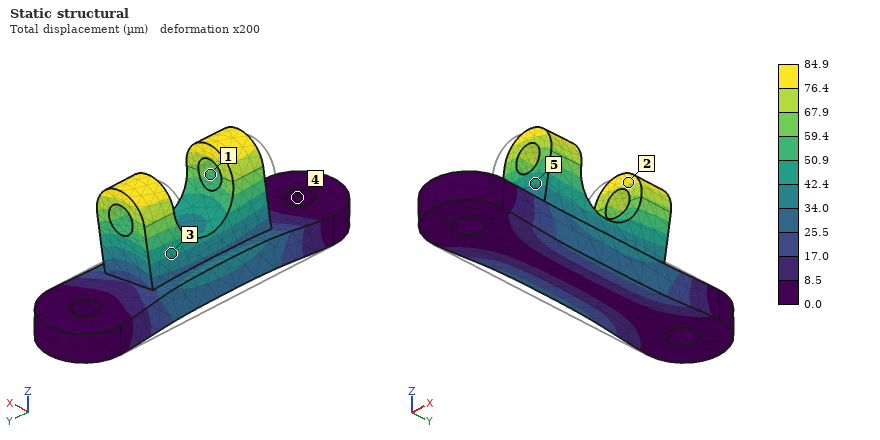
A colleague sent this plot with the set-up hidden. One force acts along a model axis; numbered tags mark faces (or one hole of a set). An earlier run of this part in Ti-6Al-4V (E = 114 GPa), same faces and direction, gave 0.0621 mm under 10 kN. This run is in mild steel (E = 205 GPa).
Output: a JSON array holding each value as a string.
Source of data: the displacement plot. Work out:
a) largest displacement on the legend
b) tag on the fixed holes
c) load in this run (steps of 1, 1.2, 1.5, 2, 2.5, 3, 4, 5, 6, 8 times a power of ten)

["84.9 µm", "4", "25 kN"]
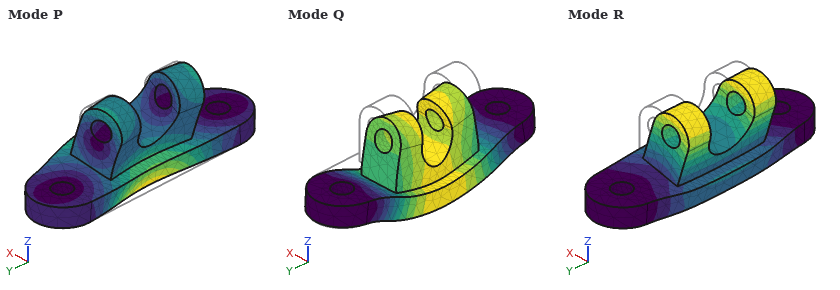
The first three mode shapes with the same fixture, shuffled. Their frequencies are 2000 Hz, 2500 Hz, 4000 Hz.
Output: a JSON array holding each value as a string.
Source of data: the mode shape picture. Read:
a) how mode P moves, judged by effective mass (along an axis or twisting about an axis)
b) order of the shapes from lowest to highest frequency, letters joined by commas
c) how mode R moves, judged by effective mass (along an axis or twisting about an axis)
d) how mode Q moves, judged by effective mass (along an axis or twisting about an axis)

["along X", "R, Q, P", "along X", "along Z"]
